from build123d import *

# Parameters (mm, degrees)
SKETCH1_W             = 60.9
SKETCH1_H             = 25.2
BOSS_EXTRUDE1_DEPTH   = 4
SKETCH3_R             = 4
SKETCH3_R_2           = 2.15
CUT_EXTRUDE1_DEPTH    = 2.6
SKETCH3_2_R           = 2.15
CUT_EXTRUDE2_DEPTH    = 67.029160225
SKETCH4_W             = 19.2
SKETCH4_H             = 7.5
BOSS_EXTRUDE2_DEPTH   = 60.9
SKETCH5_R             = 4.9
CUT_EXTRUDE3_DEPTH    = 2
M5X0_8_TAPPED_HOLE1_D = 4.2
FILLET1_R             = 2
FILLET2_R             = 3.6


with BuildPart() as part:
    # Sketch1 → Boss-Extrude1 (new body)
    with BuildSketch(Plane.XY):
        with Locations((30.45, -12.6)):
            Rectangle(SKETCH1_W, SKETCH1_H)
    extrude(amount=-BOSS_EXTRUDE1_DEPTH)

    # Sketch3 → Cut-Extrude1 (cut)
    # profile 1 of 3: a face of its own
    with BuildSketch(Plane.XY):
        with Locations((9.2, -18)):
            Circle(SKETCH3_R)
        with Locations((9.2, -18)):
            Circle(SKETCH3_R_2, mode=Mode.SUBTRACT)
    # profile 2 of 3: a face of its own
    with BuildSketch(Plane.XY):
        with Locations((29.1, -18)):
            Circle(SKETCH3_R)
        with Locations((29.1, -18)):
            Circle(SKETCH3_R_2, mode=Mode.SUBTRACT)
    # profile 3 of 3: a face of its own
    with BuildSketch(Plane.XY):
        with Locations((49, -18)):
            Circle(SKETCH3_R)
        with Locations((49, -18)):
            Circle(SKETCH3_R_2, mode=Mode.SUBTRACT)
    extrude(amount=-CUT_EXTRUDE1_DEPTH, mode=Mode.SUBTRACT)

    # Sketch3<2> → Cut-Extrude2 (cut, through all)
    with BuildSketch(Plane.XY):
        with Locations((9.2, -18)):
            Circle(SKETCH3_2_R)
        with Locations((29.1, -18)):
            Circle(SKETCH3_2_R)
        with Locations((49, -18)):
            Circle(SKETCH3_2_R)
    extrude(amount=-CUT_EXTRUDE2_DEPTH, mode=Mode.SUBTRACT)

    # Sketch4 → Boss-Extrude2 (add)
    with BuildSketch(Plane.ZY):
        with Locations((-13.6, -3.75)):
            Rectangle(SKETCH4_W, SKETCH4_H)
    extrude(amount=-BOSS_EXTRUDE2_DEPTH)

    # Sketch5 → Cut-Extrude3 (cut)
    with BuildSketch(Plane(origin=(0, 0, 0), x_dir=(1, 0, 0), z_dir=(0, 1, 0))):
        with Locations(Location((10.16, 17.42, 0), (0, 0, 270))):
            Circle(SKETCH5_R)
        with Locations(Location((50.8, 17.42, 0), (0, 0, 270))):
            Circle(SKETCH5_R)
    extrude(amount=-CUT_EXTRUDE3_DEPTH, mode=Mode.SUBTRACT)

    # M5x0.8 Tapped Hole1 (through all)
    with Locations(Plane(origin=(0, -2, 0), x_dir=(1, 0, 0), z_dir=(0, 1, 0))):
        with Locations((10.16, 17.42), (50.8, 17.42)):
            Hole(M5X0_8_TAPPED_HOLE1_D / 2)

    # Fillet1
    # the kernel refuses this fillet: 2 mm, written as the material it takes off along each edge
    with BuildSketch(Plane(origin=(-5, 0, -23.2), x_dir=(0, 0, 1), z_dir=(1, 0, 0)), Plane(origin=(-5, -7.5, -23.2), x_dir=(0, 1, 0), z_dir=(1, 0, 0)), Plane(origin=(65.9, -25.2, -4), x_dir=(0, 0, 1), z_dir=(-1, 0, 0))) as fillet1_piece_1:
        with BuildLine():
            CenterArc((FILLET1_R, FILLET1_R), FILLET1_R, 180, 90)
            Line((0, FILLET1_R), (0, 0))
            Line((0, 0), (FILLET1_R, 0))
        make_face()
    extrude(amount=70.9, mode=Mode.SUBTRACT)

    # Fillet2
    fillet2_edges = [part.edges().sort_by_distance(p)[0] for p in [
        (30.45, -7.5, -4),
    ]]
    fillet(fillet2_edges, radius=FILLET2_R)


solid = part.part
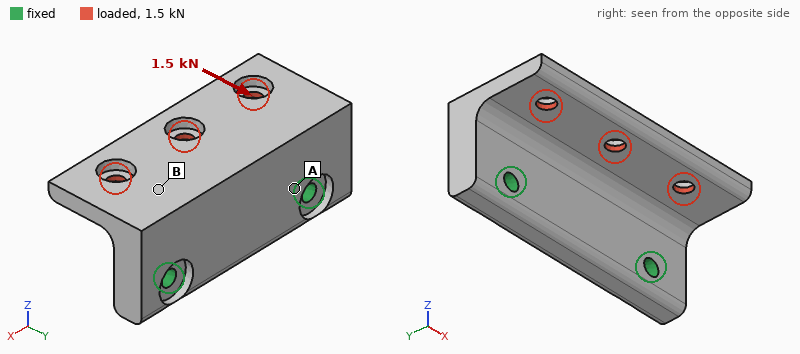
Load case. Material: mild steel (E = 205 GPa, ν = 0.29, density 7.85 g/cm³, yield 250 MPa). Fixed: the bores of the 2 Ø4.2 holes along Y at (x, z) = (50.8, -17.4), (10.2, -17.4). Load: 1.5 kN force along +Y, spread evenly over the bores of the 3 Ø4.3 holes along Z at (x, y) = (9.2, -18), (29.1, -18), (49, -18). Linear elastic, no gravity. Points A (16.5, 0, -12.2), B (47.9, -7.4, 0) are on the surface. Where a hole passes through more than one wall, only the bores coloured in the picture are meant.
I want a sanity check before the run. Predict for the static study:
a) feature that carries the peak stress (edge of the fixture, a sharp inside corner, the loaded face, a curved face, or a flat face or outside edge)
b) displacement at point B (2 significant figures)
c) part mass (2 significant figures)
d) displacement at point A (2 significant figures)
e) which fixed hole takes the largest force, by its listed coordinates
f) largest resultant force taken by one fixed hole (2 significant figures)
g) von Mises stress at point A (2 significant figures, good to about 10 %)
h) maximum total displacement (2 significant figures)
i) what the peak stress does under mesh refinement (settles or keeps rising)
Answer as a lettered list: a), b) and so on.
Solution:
a) edge of the fixture
b) 13 µm
c) 110 g
d) 5.0 µm
e) (10.2, -17.4)
f) 800 N
g) 26 MPa
h) 20 µm
i) keeps rising
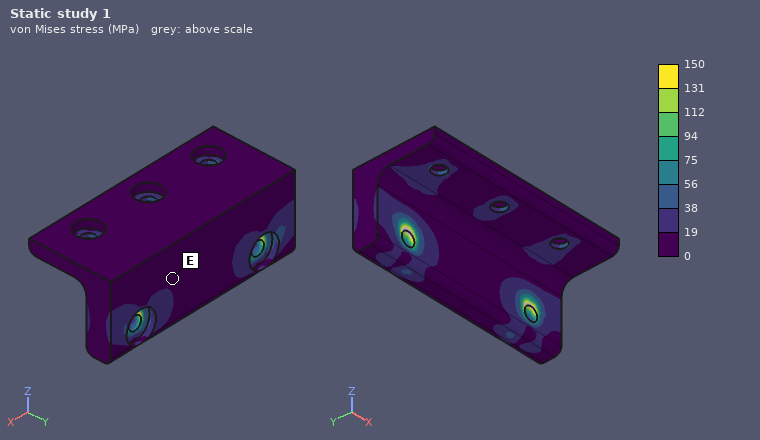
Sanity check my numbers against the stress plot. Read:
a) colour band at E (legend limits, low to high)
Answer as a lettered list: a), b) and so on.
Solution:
a) 0 to 19 MPa
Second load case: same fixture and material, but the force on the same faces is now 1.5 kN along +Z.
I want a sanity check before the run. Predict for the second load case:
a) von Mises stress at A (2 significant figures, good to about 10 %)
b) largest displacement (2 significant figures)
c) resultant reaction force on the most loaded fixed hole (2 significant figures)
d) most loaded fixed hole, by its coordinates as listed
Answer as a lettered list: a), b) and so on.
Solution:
a) 36 MPa
b) 49 µm
c) 820 N
d) (10.2, -17.4)
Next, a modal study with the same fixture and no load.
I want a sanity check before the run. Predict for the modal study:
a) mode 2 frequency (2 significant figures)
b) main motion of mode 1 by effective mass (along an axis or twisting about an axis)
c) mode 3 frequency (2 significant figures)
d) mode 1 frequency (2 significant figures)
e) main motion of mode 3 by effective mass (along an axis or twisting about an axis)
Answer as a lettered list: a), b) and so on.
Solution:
a) 8400 Hz
b) along Y
c) 12 kHz
d) 5500 Hz
e) along Y
